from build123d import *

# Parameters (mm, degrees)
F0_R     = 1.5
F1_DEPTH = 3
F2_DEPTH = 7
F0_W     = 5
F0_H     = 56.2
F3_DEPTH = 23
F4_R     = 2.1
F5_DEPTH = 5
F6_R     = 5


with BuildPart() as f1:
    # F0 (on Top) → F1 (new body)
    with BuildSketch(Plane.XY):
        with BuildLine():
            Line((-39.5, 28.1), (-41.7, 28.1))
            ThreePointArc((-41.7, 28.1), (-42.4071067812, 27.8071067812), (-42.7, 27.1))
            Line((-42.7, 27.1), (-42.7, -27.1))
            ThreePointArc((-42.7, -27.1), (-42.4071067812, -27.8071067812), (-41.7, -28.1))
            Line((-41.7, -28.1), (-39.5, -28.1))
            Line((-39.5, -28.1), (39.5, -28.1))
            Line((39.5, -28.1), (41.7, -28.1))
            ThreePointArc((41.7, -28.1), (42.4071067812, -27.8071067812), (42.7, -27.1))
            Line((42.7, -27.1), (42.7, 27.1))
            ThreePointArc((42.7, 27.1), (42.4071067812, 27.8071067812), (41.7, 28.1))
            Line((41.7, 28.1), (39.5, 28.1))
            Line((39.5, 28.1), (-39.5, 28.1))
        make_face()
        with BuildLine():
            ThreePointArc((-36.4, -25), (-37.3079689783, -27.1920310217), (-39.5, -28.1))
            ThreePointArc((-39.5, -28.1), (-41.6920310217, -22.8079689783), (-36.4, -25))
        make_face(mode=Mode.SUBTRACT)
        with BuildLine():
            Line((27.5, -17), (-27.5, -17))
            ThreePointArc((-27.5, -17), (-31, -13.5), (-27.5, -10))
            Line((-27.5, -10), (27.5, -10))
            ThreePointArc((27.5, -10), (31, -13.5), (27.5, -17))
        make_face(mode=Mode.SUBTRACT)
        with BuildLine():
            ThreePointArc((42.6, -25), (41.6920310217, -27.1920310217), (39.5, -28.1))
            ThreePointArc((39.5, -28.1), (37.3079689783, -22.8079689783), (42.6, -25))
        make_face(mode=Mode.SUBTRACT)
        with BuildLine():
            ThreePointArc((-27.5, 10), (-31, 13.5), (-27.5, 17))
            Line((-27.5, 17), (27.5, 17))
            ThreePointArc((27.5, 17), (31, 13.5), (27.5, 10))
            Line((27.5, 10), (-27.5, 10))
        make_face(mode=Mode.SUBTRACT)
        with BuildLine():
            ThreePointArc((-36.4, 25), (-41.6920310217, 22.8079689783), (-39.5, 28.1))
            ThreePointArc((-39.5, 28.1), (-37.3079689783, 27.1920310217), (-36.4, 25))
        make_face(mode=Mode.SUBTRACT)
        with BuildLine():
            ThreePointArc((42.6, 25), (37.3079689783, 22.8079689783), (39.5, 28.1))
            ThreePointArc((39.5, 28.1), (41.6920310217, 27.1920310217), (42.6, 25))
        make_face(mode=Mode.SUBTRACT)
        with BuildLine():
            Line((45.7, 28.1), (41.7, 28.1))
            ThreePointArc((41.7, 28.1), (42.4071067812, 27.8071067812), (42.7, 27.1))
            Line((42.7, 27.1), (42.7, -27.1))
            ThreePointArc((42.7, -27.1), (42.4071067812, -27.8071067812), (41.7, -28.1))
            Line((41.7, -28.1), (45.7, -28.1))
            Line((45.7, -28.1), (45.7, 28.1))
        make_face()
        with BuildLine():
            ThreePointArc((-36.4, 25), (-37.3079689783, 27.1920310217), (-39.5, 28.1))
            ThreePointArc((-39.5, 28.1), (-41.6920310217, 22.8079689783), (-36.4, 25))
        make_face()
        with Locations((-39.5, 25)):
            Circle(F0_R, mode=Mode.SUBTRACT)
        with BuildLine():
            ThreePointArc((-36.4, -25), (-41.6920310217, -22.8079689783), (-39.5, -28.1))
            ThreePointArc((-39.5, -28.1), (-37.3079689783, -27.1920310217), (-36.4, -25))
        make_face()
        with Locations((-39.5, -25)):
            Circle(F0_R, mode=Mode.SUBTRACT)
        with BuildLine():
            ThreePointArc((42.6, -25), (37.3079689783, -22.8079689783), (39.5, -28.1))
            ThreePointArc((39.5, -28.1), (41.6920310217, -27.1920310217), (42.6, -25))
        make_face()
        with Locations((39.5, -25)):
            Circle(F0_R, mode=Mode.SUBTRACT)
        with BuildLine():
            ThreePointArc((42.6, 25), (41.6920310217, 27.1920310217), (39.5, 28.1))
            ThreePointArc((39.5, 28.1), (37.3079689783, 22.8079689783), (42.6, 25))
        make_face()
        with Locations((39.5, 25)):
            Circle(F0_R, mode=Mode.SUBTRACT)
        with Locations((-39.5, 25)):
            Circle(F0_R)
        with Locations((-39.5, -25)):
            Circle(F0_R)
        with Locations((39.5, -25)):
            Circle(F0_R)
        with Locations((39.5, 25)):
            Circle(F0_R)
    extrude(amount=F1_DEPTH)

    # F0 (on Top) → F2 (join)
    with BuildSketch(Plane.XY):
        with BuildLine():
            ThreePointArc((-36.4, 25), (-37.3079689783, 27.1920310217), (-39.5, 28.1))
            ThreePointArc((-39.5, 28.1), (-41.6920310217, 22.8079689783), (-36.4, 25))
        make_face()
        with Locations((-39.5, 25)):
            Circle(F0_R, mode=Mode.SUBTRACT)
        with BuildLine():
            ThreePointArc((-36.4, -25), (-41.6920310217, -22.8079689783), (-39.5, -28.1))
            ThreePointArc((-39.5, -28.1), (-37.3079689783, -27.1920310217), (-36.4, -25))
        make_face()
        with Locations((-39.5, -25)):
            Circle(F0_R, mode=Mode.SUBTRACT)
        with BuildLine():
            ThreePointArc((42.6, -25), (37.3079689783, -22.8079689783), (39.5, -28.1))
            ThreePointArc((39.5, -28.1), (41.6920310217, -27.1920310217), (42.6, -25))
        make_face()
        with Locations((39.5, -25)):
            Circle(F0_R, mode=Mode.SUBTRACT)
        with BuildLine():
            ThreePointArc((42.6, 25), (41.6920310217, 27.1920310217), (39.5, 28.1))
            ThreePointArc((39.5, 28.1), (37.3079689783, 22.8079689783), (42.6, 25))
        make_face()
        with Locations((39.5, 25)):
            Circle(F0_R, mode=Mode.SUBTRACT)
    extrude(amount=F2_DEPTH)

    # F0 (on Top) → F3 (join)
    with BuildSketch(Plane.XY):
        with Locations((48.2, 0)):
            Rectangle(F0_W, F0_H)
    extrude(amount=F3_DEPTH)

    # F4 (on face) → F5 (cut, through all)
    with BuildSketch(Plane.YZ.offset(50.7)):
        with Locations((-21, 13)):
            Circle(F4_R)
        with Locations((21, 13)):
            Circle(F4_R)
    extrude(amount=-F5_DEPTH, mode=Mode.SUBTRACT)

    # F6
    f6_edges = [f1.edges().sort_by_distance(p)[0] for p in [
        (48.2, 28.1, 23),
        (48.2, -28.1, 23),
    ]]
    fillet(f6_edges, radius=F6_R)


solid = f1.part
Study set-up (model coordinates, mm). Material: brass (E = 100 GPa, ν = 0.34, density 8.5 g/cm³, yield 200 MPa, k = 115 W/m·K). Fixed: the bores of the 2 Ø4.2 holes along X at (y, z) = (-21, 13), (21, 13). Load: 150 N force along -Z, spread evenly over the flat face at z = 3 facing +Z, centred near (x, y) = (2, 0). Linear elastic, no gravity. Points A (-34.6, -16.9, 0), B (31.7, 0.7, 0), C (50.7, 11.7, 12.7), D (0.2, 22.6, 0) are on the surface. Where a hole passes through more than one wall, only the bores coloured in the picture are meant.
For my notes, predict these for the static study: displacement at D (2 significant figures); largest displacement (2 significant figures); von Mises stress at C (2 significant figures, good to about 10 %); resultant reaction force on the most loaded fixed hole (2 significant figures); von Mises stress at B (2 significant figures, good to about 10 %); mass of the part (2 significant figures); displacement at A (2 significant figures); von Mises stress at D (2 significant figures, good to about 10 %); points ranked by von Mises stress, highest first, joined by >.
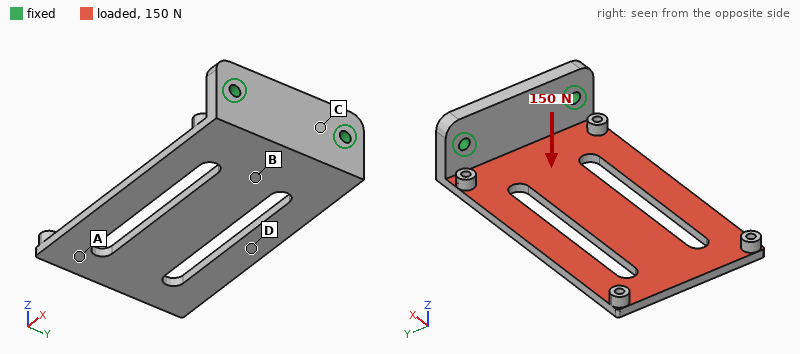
0.49 mm
1.3 mm
14 MPa
79 N
56 MPa
160 g
1.2 mm
26 MPa
B > D > C > A
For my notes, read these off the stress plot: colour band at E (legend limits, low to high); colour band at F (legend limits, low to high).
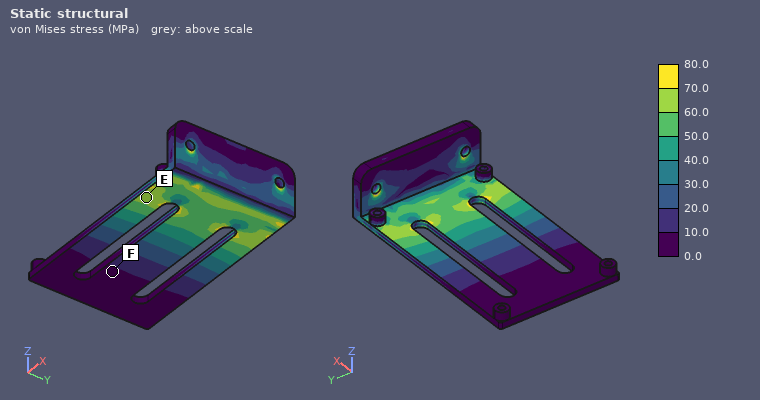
60.0 to 70.0 MPa
0.0 to 10.0 MPa
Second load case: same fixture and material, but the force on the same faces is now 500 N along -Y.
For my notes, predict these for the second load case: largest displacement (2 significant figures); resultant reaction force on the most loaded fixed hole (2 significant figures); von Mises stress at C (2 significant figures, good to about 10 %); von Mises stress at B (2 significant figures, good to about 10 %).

0.14 mm
600 N
11 MPa
11 MPa
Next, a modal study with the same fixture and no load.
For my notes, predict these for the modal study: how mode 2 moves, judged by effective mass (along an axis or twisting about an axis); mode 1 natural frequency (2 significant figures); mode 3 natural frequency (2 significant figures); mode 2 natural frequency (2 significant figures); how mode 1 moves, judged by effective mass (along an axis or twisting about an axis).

twisting about X
200 Hz
1200 Hz
630 Hz
along Z
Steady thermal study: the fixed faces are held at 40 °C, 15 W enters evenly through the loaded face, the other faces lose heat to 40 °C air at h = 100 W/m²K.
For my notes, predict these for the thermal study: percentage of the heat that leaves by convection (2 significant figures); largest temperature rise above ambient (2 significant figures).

58 %
18 K
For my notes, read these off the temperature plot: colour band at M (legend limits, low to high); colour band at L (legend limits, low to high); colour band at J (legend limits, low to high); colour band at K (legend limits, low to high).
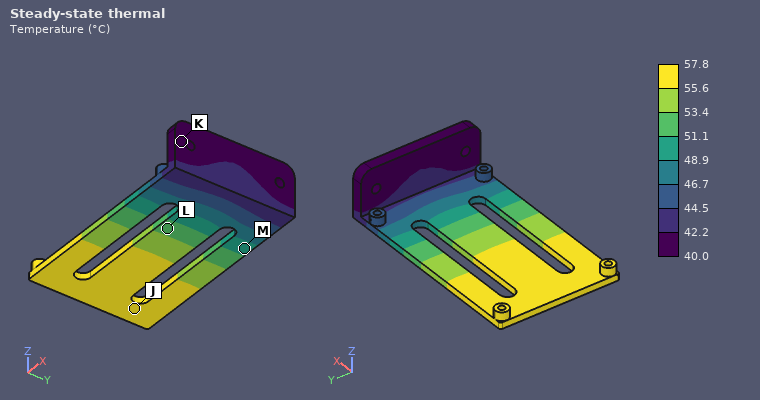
48.9 to 51.1 °C
51.1 to 53.4 °C
55.6 to 57.8 °C
40.0 to 42.2 °C
